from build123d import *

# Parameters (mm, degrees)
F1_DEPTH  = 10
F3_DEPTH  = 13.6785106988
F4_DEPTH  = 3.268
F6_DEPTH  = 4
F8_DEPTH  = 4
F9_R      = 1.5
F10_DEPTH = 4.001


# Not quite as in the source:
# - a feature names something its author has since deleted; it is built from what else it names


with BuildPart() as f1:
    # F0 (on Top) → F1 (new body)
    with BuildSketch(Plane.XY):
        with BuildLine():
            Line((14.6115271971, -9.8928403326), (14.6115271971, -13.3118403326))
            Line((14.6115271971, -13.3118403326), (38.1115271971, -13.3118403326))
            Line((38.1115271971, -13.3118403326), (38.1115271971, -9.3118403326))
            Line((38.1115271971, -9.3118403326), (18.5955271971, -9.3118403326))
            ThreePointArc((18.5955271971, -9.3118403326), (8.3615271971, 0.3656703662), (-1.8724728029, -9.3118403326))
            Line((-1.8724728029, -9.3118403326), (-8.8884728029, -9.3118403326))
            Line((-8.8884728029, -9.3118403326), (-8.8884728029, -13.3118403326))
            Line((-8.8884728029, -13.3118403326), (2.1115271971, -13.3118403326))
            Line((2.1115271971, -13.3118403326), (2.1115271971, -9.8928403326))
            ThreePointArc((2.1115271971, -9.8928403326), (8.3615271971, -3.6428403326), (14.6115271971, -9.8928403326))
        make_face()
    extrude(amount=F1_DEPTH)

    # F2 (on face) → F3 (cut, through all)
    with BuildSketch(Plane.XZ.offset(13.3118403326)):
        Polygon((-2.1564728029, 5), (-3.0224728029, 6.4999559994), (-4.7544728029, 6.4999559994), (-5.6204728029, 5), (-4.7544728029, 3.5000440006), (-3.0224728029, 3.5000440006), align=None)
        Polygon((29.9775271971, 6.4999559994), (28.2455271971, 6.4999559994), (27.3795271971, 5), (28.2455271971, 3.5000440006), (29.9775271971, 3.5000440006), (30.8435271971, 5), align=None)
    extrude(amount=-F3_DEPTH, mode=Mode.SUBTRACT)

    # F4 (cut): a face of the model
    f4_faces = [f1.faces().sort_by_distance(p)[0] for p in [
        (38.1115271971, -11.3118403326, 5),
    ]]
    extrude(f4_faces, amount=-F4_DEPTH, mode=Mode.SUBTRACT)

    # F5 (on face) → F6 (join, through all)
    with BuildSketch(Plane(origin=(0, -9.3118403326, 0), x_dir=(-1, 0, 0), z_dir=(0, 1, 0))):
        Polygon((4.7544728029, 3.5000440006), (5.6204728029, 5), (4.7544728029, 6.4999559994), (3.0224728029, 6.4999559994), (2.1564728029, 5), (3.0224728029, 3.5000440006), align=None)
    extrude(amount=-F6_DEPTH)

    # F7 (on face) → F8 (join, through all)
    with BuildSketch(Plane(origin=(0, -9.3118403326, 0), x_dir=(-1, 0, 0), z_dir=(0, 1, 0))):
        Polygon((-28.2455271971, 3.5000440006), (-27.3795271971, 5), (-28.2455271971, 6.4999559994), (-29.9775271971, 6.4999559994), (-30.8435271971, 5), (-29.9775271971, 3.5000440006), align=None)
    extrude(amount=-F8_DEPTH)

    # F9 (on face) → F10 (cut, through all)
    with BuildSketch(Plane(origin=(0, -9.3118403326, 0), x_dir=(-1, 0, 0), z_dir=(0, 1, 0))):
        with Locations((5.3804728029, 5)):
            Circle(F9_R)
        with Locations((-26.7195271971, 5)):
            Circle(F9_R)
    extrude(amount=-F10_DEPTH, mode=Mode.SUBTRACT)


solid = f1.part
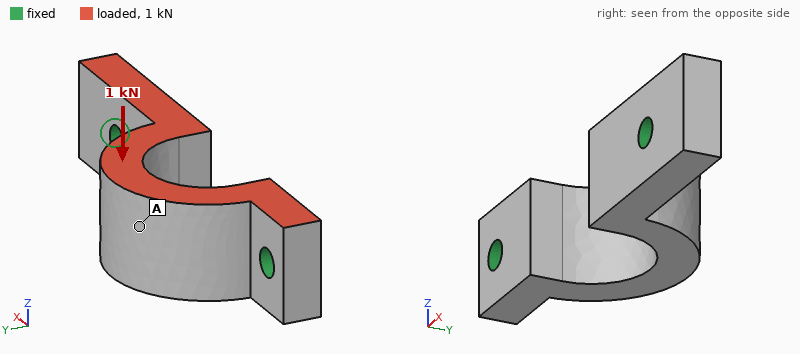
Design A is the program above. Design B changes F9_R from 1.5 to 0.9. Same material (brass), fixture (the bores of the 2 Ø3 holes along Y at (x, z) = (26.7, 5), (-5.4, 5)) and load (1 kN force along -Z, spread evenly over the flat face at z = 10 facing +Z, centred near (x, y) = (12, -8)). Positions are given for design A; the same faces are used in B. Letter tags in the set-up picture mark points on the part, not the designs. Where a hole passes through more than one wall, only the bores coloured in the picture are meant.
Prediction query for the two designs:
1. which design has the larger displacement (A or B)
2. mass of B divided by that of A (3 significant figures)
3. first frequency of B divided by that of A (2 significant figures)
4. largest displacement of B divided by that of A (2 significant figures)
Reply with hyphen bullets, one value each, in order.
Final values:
- B
- 1.02
- 0.82
- 1.5
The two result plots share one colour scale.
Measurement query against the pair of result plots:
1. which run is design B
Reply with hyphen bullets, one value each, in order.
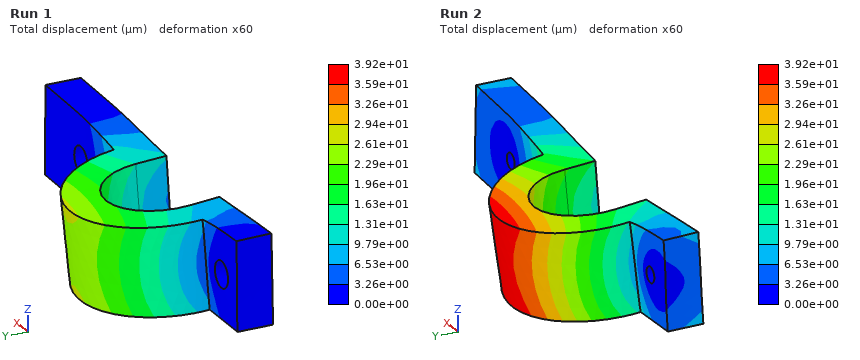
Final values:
- Run 2
